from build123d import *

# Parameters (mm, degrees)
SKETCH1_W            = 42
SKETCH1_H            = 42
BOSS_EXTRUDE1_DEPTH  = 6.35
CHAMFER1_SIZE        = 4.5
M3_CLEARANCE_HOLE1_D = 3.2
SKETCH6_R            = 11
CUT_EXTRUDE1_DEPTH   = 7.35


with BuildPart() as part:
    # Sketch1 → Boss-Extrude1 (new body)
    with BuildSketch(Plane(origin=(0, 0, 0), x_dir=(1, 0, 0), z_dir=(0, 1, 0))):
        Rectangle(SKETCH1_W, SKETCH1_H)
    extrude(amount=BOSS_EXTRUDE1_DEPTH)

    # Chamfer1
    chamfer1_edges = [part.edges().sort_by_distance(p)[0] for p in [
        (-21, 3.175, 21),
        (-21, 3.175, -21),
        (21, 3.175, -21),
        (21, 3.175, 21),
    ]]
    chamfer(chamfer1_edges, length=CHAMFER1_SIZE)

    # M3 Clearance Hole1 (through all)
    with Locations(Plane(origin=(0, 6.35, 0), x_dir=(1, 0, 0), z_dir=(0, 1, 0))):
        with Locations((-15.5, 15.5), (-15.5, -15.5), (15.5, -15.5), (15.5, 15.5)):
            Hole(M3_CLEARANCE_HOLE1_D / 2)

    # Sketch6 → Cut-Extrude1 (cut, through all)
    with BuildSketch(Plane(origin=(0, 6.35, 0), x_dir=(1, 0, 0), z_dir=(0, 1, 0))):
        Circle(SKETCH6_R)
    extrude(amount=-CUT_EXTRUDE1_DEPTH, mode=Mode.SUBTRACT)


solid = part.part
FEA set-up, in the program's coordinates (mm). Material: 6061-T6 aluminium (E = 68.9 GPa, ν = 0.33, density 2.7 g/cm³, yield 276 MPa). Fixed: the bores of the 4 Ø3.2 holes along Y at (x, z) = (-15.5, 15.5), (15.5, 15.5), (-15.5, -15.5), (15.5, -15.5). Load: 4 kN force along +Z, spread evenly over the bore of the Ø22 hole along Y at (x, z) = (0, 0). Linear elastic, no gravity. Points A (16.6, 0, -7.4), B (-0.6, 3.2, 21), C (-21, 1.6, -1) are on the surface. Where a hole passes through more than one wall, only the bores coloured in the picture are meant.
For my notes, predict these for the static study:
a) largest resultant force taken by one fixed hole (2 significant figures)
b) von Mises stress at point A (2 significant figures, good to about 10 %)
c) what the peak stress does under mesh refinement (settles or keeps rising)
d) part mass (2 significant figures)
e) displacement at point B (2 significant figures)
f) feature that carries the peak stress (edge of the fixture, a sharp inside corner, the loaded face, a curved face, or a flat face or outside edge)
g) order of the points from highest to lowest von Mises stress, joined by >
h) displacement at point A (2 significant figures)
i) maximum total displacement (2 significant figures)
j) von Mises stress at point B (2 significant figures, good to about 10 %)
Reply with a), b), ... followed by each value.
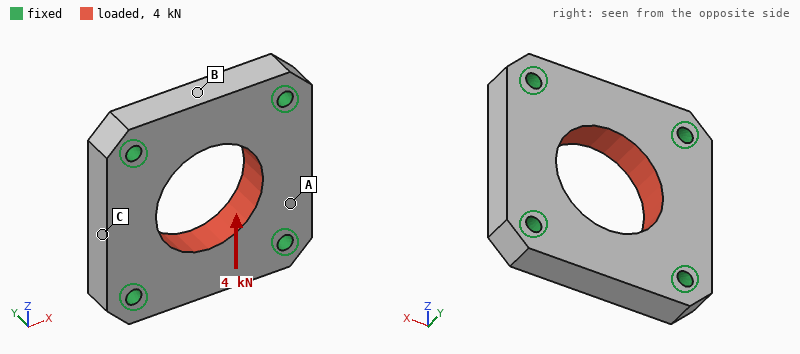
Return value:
a) 1.0 kN
b) 9.8 MPa
c) keeps rising
d) 22 g
e) 5.1 µm
f) edge of the fixture
g) B > A > C
h) 1.2 µm
i) 6.0 µm
j) 18 MPa
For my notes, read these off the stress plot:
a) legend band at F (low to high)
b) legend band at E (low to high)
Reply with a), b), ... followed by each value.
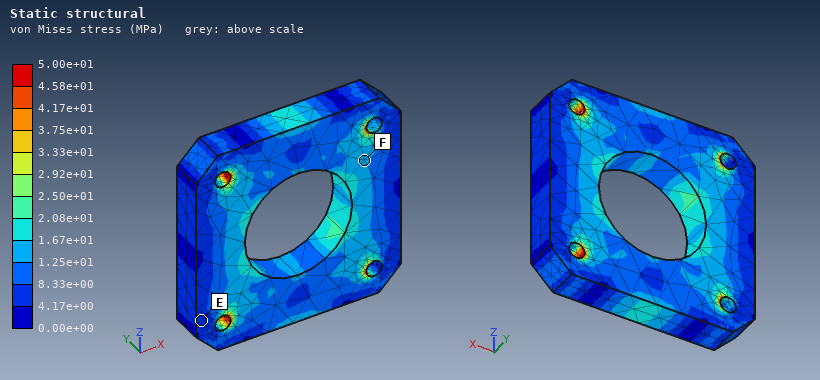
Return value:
a) 1.25e+01 to 1.67e+01 MPa
b) 4.17e+00 to 8.33e+00 MPa
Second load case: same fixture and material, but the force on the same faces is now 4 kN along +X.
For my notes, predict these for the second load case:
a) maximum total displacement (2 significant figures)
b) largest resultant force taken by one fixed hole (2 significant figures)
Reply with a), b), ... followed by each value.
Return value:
a) 6.0 µm
b) 1.0 kN
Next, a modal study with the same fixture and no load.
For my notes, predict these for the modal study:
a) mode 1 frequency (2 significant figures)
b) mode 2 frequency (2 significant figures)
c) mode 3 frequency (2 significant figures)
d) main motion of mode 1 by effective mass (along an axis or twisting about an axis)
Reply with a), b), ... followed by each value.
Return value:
a) 26 kHz
b) 28 kHz
c) 29 kHz
d) along Y
